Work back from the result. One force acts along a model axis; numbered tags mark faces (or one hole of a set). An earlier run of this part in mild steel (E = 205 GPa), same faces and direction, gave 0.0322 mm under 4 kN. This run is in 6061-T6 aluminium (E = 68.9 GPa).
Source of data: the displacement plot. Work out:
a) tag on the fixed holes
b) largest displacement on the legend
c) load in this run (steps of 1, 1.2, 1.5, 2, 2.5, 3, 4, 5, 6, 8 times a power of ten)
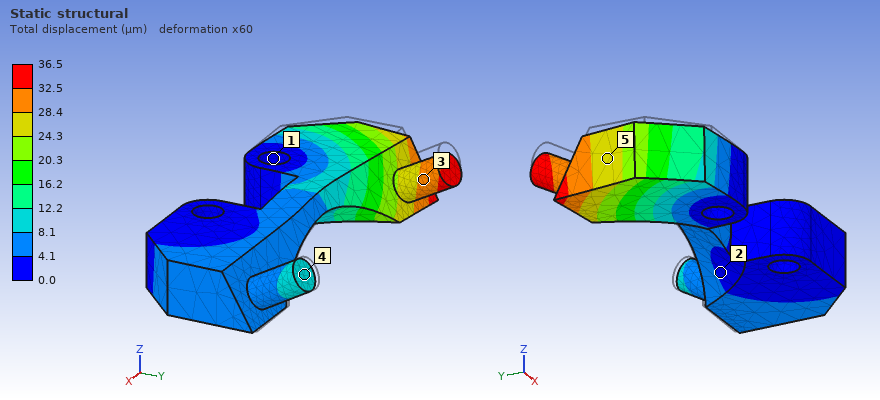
1
36.5 µm
1.5 kN
